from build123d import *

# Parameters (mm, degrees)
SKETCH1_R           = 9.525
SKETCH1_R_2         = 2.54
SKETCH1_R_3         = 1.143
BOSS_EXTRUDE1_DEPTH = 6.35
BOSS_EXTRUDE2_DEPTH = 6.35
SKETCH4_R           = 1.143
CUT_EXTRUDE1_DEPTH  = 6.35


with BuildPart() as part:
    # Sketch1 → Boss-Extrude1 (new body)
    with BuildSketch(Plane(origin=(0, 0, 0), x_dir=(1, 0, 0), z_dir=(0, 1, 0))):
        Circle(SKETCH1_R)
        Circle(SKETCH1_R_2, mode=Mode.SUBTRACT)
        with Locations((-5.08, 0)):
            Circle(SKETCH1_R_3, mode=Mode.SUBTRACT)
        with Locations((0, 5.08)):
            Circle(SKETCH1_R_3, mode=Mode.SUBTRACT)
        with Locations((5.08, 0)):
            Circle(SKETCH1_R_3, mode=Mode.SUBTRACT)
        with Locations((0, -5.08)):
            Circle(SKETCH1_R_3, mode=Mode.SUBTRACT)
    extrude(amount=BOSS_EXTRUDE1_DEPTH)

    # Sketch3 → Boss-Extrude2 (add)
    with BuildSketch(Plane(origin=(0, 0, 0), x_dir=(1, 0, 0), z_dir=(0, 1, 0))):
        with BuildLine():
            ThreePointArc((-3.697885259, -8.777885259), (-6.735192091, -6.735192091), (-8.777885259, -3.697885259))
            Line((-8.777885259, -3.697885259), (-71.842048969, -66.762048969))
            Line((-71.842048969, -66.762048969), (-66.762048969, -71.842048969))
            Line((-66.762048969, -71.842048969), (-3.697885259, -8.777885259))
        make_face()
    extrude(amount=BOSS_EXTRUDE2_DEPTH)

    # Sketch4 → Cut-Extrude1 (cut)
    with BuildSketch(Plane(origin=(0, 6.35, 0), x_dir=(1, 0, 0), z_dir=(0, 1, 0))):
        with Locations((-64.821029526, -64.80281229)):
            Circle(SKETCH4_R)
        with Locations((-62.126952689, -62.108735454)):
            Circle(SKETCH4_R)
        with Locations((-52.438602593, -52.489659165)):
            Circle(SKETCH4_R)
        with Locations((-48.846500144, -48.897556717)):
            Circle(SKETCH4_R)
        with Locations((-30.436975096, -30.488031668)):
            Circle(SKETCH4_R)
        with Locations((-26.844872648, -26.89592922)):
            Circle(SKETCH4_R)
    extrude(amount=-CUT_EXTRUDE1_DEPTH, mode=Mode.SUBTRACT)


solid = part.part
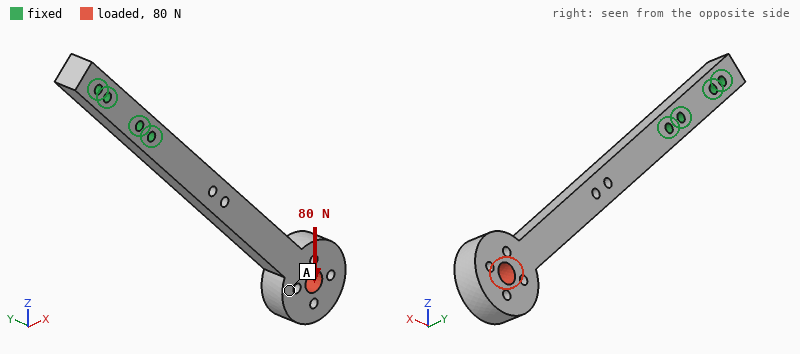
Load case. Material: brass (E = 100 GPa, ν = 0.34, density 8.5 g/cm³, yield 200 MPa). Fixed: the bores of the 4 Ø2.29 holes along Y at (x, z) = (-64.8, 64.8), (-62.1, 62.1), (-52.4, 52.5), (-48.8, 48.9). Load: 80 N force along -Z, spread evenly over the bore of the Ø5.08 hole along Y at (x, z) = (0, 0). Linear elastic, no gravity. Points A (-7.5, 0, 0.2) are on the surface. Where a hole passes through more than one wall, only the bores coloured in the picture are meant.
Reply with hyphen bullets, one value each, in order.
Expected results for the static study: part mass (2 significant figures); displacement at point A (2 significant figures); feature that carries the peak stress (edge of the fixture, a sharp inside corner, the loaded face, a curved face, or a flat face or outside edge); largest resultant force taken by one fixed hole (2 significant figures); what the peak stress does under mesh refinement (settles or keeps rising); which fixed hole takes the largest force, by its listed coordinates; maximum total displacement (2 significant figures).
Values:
- 46 g
- 0.31 mm
- edge of the fixture
- 380 N
- keeps rising
- (-48.8, 48.9)
- 0.42 mm
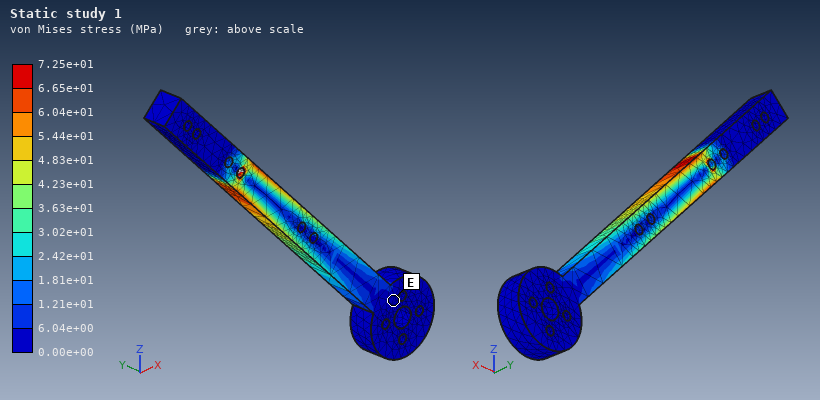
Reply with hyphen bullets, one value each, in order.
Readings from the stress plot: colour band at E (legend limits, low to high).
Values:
- 0.00e+00 to 6.04e+00 MPa
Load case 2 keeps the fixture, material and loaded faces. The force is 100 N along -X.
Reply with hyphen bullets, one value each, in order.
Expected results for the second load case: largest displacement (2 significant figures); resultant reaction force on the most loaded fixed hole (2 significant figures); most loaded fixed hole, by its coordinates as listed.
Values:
- 0.52 mm
- 470 N
- (-48.8, 48.9)
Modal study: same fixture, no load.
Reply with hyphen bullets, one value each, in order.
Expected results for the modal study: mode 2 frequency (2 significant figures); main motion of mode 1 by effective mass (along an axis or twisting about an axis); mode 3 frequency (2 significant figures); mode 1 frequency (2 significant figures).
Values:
- 490 Hz
- along Y
- 3100 Hz
- 440 Hz
